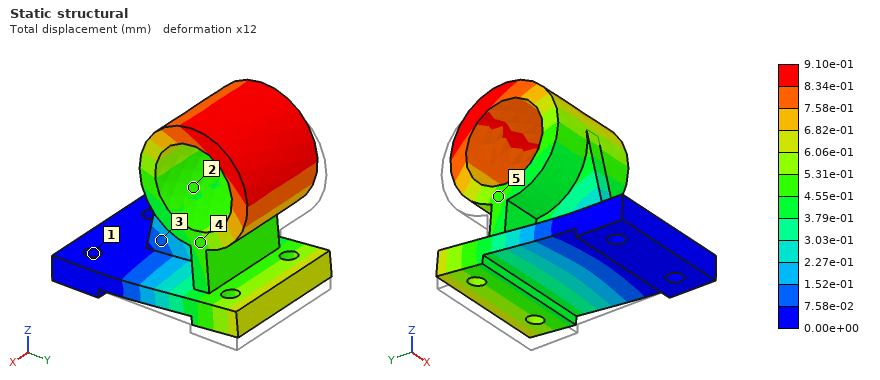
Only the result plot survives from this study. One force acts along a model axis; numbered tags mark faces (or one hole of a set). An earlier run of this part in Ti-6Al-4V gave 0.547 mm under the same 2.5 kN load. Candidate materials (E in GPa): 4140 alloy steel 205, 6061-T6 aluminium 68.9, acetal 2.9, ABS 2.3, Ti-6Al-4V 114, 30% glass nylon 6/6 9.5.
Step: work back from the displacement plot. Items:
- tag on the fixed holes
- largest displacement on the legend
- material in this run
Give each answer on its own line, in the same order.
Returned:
1
9.10e-01 mm
6061-T6 aluminium
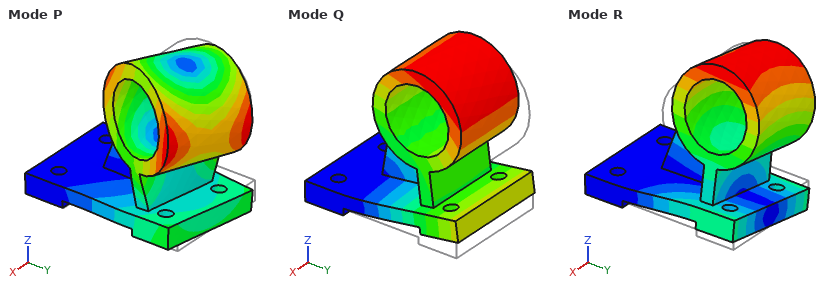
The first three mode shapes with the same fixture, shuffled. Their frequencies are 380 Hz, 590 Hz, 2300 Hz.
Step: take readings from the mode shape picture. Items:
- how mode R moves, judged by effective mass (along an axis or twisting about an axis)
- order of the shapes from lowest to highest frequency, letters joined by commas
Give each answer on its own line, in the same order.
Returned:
along X
Q, R, P
